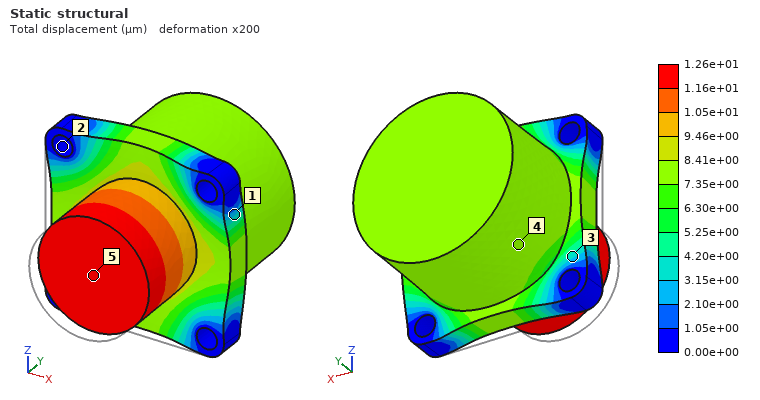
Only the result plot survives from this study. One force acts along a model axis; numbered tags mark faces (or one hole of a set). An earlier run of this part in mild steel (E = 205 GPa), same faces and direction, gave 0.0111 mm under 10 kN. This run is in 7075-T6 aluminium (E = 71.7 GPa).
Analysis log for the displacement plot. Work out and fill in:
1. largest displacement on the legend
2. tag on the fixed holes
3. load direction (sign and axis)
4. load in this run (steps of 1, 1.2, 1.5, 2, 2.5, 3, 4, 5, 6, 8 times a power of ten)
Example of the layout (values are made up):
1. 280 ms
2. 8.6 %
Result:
1. 1.26e+01 µm
2. 2
3. +Y
4. 4 kN
